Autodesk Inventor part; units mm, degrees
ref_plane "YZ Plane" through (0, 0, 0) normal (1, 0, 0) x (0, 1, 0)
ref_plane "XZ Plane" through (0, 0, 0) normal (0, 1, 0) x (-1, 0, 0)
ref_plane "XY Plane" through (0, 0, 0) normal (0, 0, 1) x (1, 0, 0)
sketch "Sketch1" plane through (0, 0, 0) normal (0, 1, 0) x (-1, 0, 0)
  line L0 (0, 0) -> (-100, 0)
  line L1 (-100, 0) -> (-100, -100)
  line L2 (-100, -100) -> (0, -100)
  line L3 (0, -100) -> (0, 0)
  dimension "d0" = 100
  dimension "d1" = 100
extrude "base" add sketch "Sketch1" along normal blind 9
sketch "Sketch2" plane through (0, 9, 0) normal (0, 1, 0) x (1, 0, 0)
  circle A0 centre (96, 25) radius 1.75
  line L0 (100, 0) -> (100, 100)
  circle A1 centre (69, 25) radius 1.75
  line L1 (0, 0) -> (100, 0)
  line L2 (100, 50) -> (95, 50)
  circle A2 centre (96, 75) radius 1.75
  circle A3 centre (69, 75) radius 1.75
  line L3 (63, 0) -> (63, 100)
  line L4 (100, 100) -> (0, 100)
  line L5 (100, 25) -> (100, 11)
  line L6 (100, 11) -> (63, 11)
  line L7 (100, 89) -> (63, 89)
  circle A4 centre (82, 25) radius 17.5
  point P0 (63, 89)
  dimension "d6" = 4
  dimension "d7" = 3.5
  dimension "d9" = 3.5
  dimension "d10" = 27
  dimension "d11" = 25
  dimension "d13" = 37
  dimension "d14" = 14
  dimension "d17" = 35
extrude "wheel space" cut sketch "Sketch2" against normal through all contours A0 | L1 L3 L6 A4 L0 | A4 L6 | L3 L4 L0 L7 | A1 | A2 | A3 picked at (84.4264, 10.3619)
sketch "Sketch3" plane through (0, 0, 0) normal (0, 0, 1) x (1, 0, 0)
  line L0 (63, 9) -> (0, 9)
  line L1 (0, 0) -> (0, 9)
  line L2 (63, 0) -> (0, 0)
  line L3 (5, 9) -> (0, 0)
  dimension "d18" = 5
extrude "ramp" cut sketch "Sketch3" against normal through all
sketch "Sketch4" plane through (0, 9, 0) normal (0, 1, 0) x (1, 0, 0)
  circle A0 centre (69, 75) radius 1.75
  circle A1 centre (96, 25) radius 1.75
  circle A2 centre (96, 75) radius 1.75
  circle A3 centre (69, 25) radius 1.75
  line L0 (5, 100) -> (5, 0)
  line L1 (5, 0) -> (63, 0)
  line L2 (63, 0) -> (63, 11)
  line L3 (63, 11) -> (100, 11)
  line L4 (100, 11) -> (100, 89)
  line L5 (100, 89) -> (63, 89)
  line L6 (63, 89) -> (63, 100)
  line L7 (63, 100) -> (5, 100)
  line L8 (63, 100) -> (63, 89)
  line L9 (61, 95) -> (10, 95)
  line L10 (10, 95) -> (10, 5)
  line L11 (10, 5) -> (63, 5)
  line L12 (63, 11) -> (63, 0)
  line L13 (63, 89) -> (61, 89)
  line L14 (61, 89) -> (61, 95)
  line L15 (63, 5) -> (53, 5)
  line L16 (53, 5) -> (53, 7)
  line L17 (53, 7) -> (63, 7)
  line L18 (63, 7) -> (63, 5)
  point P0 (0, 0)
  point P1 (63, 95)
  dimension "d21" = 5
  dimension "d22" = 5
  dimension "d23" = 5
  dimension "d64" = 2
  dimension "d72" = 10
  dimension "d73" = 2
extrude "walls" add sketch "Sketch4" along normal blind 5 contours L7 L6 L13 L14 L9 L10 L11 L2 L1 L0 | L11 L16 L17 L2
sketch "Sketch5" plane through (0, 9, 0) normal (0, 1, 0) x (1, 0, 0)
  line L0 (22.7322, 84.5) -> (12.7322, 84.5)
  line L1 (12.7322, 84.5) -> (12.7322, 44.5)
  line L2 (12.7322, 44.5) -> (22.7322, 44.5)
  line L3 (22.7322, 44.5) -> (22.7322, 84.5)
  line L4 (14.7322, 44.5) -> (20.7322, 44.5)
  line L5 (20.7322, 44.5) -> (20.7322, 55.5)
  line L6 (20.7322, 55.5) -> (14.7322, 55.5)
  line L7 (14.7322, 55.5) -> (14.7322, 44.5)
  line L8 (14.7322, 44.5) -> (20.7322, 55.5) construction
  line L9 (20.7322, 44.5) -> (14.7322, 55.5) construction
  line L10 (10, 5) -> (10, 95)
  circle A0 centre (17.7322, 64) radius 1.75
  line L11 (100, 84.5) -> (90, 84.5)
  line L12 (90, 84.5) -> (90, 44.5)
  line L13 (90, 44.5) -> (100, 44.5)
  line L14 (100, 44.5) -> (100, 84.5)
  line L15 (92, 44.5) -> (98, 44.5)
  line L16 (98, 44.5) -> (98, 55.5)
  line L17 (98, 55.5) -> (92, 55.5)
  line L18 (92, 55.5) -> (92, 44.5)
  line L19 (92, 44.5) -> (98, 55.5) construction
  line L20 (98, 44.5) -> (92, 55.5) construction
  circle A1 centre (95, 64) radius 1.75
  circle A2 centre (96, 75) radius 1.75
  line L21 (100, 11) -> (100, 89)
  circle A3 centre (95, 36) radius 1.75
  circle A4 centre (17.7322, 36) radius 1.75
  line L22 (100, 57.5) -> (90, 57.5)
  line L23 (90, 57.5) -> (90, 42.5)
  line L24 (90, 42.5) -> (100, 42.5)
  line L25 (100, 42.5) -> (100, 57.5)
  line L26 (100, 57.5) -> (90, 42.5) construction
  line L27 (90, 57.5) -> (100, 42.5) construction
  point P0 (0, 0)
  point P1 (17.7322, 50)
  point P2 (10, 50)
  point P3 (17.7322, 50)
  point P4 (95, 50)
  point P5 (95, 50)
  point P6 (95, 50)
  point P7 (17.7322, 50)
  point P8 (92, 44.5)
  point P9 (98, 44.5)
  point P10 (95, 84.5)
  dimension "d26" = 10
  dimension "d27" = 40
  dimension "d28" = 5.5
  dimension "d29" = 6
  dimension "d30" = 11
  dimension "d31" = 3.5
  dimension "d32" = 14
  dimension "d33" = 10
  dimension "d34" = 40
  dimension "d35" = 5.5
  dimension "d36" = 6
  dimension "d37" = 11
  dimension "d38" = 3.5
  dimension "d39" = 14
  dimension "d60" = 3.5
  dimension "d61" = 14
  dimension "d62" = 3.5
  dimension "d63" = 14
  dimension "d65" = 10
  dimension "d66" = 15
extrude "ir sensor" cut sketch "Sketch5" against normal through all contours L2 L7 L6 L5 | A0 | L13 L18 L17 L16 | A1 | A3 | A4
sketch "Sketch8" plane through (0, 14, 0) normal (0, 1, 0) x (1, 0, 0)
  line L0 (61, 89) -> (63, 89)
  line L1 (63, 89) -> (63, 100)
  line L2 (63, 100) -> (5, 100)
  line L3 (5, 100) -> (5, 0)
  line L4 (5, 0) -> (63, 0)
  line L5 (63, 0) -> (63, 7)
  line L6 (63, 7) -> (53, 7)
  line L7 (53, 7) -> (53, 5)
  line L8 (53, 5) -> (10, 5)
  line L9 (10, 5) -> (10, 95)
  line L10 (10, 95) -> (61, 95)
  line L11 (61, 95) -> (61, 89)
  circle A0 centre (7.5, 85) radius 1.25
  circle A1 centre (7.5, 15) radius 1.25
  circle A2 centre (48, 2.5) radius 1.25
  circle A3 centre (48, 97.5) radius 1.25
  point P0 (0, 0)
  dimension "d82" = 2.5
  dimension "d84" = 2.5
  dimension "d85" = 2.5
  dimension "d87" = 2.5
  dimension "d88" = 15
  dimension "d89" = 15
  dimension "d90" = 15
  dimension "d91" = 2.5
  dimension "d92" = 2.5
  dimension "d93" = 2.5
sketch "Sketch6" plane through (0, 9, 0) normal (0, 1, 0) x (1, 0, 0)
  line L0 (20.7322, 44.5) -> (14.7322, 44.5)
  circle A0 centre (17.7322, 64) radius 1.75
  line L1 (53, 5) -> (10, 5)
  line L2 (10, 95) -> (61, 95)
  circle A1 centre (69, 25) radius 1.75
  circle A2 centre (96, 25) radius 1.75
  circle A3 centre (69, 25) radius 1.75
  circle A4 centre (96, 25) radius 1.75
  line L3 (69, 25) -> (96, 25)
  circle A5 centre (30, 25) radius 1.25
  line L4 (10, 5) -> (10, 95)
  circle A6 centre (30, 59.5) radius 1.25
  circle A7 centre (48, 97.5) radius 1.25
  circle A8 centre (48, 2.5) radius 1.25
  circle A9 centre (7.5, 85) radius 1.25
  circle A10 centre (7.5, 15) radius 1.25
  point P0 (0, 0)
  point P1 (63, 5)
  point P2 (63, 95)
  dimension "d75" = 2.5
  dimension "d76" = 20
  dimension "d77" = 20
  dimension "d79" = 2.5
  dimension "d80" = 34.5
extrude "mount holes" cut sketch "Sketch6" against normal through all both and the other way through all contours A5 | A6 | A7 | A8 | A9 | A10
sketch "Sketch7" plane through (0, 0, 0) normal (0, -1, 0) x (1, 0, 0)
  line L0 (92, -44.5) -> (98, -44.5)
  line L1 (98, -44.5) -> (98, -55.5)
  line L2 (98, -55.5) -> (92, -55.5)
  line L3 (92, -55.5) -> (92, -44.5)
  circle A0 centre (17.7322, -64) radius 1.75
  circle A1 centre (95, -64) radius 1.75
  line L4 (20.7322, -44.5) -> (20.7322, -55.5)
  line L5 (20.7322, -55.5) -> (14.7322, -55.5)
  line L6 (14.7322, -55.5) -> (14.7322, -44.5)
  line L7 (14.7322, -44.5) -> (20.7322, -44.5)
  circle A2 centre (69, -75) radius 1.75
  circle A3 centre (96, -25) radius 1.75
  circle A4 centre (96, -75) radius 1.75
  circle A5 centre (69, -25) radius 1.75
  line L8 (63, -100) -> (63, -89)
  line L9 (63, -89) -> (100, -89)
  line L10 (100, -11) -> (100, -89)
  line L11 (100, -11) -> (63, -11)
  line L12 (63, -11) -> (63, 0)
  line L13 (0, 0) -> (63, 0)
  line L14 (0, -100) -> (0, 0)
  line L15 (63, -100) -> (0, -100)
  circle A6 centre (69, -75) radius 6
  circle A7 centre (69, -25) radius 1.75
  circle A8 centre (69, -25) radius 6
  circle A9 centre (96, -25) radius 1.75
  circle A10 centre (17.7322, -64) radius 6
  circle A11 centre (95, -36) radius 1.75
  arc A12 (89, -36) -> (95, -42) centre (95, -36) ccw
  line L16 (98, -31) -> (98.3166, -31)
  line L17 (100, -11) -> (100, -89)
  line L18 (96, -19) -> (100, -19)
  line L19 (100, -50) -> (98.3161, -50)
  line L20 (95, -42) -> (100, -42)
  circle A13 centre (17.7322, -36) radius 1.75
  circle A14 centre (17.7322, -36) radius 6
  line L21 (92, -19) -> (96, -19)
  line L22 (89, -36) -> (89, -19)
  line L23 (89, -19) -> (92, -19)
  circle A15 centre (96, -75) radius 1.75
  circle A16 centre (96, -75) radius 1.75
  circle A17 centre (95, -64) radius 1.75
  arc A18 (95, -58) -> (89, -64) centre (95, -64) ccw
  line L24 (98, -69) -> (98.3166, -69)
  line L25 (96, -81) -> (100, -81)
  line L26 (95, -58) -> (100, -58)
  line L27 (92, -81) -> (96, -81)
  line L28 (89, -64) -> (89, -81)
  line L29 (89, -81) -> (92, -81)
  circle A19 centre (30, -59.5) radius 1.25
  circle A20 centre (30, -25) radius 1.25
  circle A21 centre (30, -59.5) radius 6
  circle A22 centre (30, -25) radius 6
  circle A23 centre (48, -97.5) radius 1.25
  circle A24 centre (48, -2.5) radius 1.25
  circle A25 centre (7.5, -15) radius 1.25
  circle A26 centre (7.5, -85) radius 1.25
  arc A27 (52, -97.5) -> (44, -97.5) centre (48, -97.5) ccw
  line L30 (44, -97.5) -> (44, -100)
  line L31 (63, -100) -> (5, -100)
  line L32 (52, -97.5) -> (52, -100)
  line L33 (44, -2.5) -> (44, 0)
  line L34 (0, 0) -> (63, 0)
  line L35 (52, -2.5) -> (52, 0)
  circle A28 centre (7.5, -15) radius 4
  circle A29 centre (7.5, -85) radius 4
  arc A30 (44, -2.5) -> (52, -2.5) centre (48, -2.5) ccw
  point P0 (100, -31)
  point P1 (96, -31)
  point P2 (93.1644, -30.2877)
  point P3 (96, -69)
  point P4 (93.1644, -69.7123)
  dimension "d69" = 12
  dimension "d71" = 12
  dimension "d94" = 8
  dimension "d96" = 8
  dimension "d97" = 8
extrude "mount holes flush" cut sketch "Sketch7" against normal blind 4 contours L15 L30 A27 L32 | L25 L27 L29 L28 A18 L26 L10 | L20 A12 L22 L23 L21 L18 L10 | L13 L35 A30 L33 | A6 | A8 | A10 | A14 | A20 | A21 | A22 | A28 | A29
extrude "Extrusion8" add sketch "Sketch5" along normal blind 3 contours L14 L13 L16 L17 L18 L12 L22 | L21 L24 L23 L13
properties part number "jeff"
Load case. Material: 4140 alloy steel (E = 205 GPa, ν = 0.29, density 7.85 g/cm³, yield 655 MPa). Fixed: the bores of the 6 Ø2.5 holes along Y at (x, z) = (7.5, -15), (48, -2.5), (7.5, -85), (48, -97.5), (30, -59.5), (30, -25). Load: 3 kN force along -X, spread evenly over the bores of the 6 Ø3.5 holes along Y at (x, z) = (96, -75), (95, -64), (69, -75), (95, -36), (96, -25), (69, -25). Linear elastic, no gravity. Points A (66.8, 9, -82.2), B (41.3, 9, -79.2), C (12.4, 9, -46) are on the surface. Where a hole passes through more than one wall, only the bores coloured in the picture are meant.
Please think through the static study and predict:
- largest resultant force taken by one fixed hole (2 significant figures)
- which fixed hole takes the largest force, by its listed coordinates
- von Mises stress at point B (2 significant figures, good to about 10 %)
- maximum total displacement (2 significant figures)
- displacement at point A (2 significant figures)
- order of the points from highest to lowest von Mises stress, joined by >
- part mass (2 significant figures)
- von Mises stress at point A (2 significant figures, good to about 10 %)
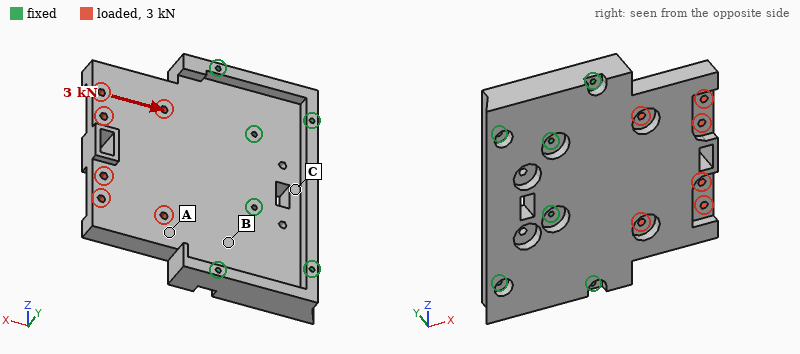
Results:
800 N
(30, -59.5)
4.5 MPa
8.6 µm
1.9 µm
A > B > C
620 g
10 MPa
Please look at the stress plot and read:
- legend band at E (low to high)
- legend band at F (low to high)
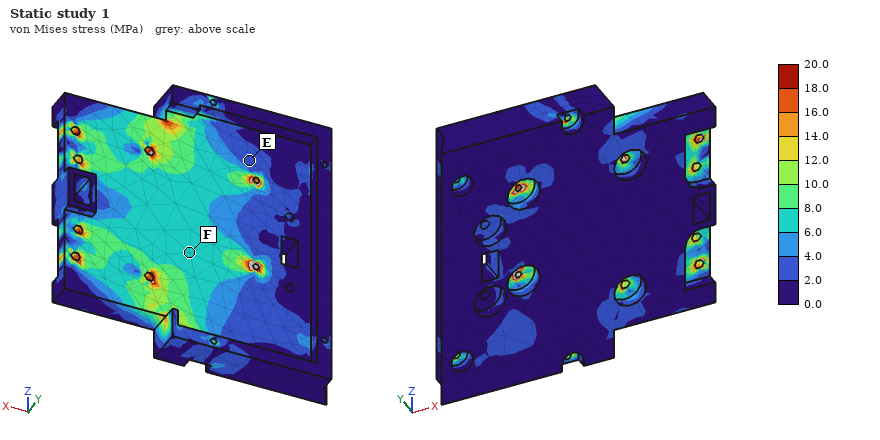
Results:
2.0 to 4.0 MPa
6.0 to 8.0 MPa
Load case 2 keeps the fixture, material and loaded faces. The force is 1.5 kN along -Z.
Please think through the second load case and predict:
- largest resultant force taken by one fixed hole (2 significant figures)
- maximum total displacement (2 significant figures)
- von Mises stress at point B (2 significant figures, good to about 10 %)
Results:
720 N
4.0 µm
1.7 MPa
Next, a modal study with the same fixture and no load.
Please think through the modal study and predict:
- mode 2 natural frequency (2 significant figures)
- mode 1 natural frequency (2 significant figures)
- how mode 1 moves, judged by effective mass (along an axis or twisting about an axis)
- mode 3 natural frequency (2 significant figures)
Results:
4400 Hz
2000 Hz
along Y
8200 Hz
